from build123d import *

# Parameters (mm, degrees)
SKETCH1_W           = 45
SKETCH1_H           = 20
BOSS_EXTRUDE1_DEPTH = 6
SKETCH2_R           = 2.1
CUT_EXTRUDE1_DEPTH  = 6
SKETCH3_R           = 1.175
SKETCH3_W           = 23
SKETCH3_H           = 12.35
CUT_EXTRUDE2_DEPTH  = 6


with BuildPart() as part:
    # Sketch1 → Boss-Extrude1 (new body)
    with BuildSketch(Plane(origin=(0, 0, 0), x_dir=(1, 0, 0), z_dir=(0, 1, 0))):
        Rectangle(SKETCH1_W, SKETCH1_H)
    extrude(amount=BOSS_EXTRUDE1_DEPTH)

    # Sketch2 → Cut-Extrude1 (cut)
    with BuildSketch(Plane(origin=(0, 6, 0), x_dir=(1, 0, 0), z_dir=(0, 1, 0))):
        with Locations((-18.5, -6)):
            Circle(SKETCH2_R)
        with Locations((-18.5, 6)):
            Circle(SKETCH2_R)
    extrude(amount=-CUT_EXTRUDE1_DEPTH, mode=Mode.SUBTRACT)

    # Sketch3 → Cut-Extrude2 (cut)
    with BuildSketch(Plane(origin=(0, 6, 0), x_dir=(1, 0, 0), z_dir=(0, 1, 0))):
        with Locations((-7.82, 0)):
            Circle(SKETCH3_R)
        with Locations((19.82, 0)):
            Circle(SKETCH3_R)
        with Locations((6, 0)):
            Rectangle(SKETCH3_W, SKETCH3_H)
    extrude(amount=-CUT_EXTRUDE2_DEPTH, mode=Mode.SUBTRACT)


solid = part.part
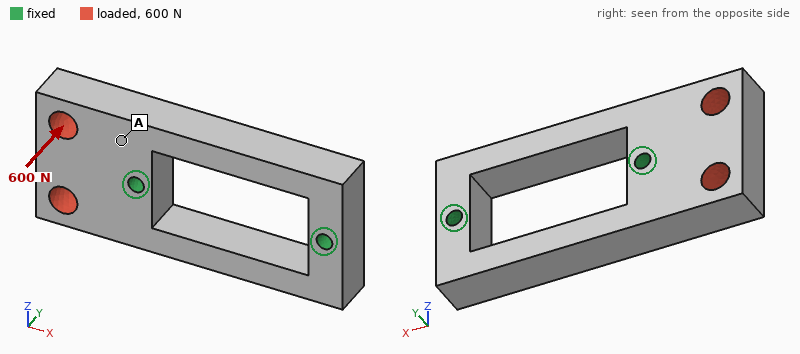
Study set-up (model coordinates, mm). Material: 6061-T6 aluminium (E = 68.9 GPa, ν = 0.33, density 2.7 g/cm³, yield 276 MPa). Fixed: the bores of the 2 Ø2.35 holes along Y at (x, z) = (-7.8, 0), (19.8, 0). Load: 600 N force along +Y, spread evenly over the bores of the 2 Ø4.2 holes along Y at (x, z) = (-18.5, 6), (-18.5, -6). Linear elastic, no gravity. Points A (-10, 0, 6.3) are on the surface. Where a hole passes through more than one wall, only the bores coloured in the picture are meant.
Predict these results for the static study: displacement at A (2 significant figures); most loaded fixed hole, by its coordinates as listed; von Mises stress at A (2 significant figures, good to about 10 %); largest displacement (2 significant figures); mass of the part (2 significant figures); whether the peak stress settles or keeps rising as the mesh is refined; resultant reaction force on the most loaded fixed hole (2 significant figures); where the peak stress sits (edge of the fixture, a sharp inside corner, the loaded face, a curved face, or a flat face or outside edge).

5.9 µm
(-7.8, 0)
23 MPa
30 µm
9.4 g
keeps rising
650 N
edge of the fixture
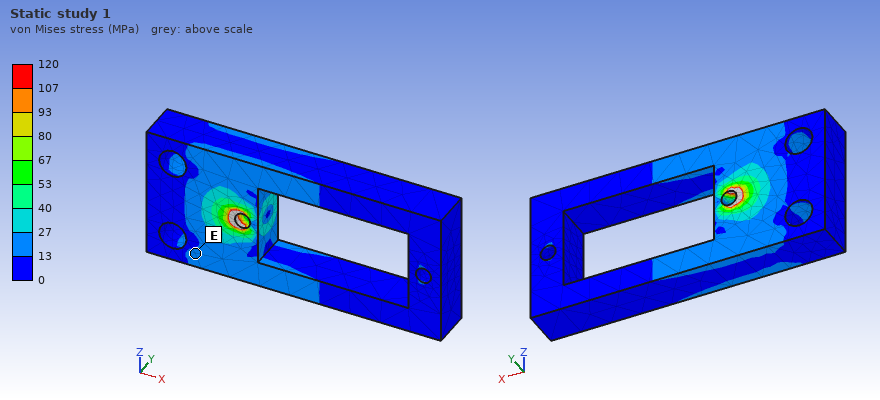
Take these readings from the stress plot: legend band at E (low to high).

13 to 27 MPa
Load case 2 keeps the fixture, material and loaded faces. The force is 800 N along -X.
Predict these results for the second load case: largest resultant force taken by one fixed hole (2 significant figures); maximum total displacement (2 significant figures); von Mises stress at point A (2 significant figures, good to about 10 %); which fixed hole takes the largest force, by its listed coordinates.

730 N
3.3 µm
4.0 MPa
(-7.8, 0)
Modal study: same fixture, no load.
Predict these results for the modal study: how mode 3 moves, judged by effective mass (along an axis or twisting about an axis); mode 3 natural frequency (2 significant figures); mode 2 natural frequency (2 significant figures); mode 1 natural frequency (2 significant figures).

twisting about X
19 kHz
16 kHz
14 kHz
